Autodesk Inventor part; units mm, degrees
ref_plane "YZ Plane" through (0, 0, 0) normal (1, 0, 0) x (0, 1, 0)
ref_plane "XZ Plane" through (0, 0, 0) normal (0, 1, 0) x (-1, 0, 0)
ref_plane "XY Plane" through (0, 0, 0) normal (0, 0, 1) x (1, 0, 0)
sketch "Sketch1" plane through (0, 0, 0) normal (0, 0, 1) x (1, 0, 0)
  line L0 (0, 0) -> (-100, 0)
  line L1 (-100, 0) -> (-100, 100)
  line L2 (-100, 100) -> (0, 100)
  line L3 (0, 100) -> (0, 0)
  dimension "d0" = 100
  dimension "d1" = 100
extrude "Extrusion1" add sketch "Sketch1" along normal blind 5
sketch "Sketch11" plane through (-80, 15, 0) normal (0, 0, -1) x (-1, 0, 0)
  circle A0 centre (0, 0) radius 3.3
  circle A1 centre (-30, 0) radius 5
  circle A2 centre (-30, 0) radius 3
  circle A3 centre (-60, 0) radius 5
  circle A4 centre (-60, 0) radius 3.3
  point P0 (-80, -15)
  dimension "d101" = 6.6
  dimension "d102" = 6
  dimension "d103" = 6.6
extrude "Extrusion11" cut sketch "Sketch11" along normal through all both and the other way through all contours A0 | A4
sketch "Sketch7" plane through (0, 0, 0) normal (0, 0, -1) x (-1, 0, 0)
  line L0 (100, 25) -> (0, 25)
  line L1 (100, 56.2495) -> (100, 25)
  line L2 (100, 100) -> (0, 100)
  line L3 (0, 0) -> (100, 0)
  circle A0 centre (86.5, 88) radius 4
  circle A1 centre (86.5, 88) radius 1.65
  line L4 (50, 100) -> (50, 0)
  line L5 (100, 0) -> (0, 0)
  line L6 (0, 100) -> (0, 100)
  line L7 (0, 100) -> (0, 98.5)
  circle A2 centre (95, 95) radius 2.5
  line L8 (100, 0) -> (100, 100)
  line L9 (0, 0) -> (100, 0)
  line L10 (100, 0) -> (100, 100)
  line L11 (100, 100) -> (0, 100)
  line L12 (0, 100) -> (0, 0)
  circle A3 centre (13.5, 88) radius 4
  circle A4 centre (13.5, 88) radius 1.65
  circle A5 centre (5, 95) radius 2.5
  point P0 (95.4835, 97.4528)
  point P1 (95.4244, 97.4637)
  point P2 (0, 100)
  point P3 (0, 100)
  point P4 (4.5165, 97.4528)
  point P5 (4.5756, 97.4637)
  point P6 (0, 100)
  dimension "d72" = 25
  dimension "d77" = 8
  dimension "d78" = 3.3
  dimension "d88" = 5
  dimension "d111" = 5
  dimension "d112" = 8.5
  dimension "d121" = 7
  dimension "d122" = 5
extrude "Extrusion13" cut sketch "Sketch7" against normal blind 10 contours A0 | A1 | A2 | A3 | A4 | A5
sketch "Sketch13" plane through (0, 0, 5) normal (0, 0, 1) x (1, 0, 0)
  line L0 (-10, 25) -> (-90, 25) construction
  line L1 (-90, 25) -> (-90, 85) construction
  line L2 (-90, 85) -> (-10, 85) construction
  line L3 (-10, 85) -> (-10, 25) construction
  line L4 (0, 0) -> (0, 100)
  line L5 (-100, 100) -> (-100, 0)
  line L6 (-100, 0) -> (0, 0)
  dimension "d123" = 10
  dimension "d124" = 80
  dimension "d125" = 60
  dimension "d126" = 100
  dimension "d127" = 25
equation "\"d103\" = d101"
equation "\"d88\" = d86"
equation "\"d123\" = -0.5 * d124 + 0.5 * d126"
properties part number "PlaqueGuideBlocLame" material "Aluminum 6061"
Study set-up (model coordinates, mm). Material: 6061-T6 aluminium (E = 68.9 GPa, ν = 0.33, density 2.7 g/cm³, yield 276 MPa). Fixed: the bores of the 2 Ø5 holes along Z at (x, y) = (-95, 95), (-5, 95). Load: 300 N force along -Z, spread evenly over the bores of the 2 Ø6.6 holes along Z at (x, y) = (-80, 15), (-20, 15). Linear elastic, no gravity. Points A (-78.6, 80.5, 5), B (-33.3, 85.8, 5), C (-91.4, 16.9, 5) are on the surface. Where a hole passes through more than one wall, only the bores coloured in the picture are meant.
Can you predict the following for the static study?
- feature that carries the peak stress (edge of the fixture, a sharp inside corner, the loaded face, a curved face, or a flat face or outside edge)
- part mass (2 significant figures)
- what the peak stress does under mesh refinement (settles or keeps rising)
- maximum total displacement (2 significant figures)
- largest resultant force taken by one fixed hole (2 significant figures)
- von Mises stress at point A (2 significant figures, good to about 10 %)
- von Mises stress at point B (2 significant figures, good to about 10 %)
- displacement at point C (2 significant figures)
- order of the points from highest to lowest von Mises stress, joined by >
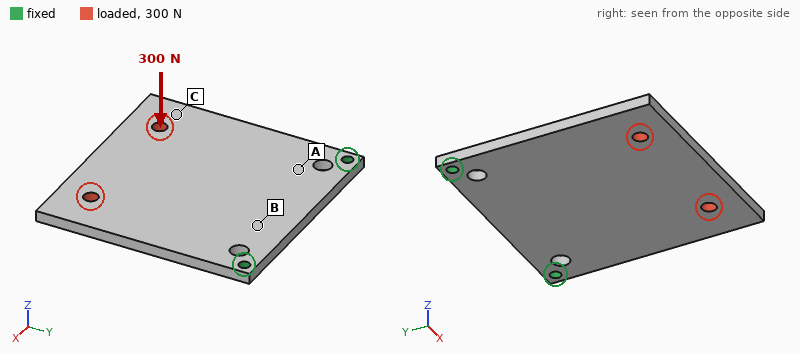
edge of the fixture
130 g
keeps rising
1.7 mm
150 N
52 MPa
35 MPa
1.3 mm
A > B > C
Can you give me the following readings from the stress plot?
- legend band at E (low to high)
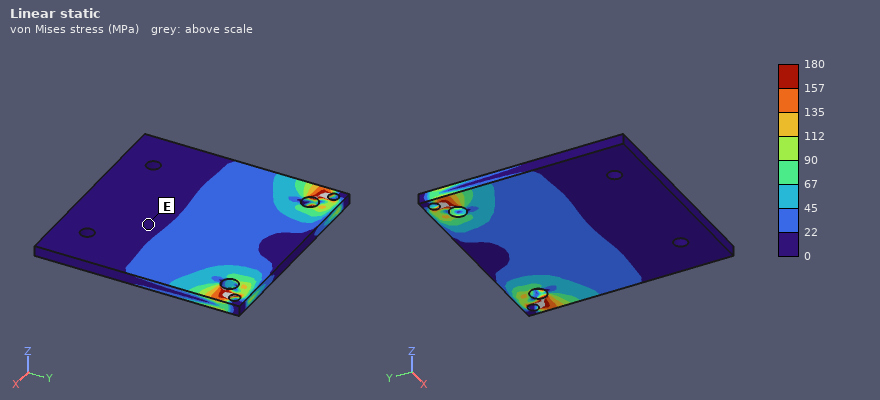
0 to 22 MPa
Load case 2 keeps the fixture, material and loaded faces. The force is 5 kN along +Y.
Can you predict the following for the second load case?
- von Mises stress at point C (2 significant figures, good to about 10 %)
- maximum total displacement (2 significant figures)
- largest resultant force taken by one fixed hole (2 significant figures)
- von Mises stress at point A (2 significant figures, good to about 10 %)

8.1 MPa
28 µm
2.6 kN
9.4 MPa
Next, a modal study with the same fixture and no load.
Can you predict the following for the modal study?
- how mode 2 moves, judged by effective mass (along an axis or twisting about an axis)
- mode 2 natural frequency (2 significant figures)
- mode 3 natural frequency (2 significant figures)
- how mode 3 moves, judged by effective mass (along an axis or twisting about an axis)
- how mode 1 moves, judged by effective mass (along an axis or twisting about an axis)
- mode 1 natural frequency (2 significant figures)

twisting about Y
1000 Hz
2200 Hz
along Z
along Z
320 Hz
